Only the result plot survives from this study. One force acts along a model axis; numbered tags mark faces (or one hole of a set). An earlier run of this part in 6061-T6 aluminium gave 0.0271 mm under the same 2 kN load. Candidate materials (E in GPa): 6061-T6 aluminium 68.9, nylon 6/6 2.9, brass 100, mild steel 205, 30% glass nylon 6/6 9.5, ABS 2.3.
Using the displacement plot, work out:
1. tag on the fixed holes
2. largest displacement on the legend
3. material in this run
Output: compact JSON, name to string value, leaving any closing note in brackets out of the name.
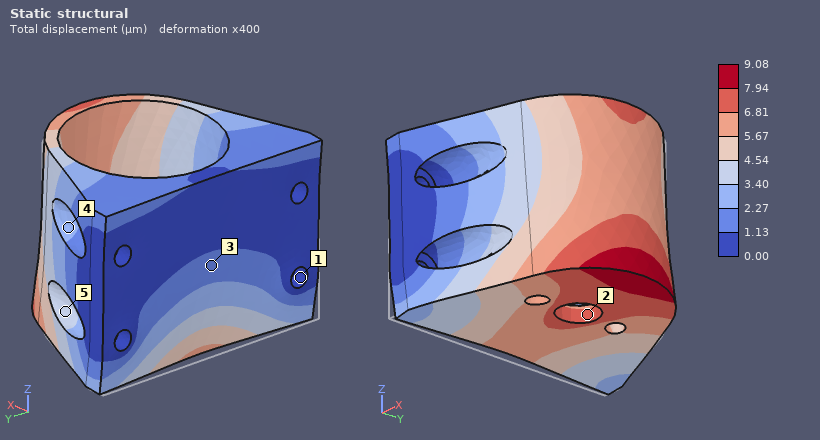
{"tag on the fixed holes": "1", "largest displacement on the legend": "9.08 µm", "material in this run": "mild steel"}
